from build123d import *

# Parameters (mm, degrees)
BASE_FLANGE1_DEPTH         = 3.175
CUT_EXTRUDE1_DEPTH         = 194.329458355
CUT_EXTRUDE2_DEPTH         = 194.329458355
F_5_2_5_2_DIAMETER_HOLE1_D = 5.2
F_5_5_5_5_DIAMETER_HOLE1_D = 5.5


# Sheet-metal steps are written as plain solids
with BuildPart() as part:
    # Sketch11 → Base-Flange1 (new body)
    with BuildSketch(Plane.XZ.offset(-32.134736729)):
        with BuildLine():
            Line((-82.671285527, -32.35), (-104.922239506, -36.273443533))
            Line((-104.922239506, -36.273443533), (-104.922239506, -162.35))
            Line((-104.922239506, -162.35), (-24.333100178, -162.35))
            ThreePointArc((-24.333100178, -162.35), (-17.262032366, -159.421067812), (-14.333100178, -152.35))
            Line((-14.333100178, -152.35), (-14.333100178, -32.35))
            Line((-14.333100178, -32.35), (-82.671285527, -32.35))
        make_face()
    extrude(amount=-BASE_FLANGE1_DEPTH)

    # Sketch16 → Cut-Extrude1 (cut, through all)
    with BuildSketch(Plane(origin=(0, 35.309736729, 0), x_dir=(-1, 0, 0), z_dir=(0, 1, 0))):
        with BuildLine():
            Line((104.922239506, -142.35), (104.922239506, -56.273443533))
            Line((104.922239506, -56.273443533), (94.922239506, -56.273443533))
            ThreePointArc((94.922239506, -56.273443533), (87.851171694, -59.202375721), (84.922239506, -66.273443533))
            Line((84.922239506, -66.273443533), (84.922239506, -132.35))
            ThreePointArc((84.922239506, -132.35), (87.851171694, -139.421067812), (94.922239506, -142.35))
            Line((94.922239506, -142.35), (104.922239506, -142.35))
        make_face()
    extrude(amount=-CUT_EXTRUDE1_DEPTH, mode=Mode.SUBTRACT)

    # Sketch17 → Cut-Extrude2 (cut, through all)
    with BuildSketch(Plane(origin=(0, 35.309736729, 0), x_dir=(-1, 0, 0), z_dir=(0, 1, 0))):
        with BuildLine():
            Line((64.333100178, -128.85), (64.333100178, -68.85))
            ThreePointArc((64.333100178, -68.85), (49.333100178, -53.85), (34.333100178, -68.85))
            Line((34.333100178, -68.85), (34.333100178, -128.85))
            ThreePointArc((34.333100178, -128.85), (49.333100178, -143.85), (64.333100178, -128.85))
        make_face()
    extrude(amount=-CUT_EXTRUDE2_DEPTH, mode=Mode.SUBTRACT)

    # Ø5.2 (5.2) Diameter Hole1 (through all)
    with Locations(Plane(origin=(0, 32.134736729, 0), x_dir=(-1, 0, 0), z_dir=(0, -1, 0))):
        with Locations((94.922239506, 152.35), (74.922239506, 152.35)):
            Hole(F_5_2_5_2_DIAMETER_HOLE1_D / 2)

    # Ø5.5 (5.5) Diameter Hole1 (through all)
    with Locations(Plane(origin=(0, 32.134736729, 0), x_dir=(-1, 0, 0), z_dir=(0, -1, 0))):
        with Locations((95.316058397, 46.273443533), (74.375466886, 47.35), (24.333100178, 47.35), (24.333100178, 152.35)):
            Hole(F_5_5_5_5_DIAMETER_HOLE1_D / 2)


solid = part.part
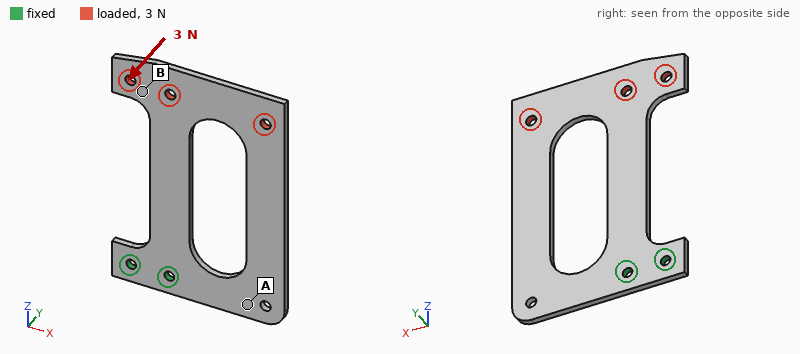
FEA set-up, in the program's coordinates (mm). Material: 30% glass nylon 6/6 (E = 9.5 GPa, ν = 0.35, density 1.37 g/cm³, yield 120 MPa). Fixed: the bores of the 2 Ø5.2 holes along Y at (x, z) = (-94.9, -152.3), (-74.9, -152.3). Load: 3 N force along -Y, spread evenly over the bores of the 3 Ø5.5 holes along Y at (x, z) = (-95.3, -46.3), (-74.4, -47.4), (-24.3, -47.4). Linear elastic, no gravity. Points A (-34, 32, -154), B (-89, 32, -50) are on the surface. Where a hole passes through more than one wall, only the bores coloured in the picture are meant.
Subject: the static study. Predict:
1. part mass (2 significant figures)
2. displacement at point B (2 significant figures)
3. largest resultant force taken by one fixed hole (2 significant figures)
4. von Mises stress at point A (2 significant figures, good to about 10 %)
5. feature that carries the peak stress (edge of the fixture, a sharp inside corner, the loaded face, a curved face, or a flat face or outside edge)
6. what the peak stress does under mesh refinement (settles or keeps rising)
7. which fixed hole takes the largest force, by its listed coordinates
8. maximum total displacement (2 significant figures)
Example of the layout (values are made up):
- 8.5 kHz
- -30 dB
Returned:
- 32 g
- 1.2 mm
- 4.7 N
- 1.7 MPa
- edge of the fixture
- keeps rising
- (-74.9, -152.3)
- 1.6 mm
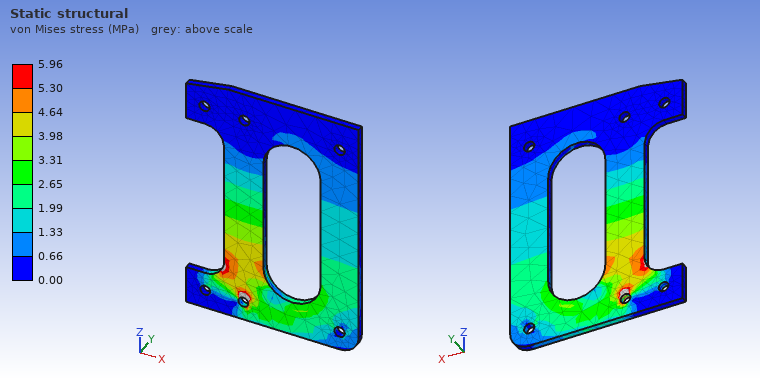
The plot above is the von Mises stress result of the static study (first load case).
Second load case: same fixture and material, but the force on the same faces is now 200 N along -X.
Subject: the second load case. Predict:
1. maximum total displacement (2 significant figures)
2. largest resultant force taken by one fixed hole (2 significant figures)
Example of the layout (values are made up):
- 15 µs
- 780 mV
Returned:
- 1.8 mm
- 900 N
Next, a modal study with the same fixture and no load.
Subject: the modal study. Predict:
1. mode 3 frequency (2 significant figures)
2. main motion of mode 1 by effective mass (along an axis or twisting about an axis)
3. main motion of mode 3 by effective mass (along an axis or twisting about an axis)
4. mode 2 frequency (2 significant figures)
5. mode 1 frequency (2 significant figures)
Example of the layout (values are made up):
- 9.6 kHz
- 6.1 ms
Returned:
- 380 Hz
- along Y
- along Y
- 170 Hz
- 66 Hz
